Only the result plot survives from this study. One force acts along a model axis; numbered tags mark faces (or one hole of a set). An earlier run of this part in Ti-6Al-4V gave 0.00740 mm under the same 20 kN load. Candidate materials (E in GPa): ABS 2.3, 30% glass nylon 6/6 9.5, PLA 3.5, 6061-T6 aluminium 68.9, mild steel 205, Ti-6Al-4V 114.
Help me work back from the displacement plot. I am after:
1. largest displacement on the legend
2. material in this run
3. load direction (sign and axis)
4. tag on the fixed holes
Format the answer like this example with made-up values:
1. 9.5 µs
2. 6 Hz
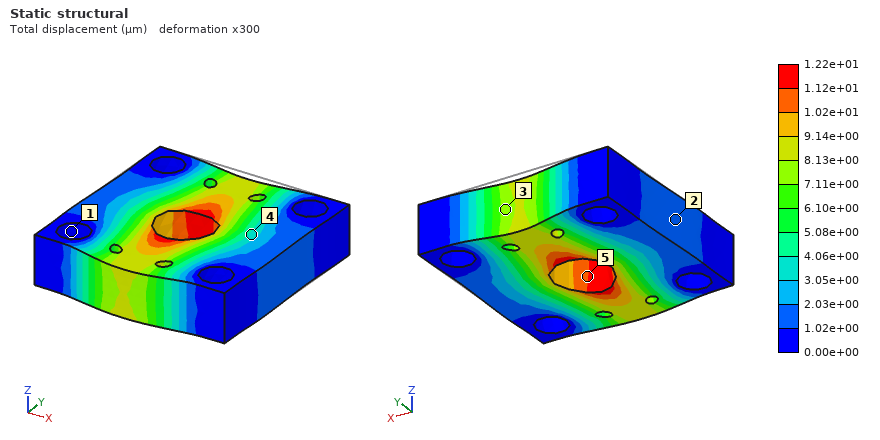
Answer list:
1. 1.22e+01 µm
2. 6061-T6 aluminium
3. -Y
4. 1
